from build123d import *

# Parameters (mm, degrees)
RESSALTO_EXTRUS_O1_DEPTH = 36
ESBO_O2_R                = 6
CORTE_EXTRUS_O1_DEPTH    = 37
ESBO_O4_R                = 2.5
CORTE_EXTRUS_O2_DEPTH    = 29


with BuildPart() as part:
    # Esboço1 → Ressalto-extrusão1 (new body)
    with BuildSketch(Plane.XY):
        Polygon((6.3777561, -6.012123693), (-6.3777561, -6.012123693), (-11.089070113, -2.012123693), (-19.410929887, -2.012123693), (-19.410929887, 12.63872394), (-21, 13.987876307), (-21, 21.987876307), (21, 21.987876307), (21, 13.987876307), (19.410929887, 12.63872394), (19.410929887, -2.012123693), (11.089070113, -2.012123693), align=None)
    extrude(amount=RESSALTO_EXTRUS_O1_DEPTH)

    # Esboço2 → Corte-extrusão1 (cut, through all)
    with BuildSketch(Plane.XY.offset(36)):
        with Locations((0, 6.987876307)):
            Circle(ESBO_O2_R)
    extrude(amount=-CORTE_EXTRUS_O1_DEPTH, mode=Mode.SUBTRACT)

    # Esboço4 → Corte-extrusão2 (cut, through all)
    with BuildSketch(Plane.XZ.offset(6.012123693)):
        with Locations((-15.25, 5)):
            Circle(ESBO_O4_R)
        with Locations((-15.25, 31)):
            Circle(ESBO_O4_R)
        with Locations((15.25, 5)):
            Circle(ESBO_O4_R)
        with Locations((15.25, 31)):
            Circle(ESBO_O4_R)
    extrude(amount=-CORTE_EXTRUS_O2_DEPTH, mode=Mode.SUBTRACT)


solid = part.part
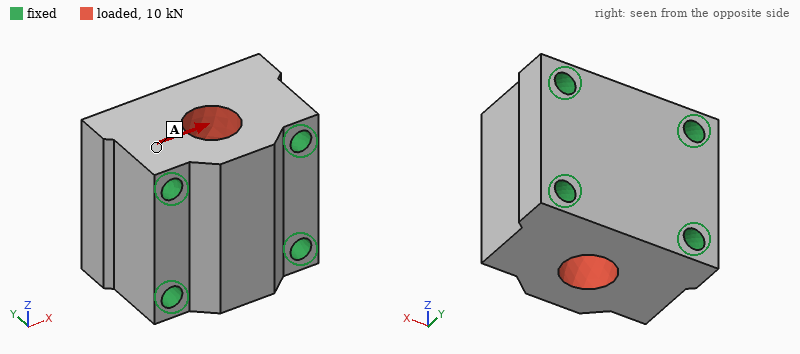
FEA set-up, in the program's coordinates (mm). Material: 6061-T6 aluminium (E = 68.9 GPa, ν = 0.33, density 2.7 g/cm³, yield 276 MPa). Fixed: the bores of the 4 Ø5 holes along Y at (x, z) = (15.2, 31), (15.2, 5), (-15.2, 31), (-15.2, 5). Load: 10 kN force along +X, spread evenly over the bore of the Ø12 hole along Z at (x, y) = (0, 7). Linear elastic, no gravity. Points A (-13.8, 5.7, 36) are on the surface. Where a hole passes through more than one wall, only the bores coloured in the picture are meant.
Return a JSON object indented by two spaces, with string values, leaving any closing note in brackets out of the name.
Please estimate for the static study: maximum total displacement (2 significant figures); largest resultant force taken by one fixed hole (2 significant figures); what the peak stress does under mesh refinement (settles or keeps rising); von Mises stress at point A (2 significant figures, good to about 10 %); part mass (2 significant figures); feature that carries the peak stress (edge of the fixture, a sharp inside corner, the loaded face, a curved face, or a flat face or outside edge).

{
  "maximum total displacement": "2.5 µm",
  "largest resultant force taken by one fixed hole": "2.6 kN",
  "what the peak stress does under mesh refinement": "keeps rising",
  "von Mises stress at point A": "4.1 MPa",
  "part mass": "84 g",
  "feature that carries the peak stress": "edge of the fixture"
}
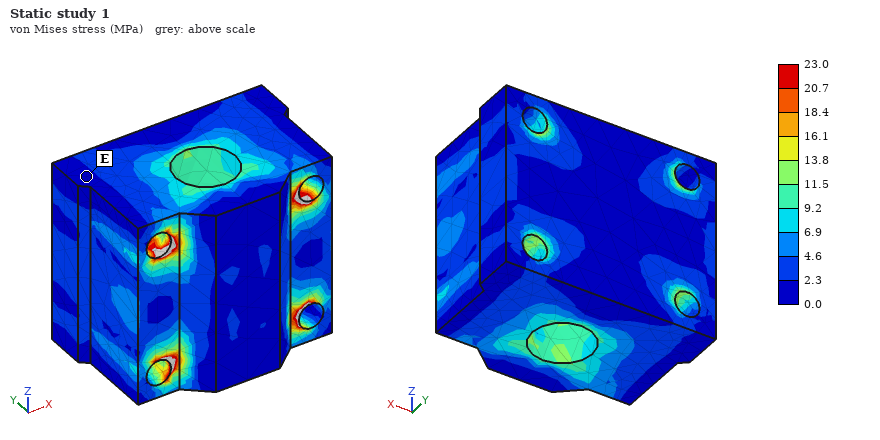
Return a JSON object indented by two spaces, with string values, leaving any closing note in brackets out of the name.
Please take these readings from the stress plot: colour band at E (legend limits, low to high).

{
  "colour band at E": "0.0 to 2.3 MPa"
}
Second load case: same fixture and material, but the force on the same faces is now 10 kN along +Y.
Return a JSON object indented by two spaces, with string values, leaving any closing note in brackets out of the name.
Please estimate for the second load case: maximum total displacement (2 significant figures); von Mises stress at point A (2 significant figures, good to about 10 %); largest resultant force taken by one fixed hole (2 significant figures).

{
  "maximum total displacement": "4.4 µm",
  "von Mises stress at point A": "7.1 MPa",
  "largest resultant force taken by one fixed hole": "2.5 kN"
}
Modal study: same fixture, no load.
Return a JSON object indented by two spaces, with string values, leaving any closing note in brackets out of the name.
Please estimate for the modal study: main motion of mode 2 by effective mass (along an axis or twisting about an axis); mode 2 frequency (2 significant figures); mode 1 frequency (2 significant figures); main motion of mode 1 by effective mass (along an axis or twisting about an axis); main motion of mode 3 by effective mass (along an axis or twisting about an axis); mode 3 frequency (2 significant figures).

{
  "main motion of mode 2 by effective mass": "along Z",
  "mode 2 frequency": "45 kHz",
  "mode 1 frequency": "43 kHz",
  "main motion of mode 1 by effective mass": "along Y",
  "main motion of mode 3 by effective mass": "along Z",
  "mode 3 frequency": "51 kHz"
}
